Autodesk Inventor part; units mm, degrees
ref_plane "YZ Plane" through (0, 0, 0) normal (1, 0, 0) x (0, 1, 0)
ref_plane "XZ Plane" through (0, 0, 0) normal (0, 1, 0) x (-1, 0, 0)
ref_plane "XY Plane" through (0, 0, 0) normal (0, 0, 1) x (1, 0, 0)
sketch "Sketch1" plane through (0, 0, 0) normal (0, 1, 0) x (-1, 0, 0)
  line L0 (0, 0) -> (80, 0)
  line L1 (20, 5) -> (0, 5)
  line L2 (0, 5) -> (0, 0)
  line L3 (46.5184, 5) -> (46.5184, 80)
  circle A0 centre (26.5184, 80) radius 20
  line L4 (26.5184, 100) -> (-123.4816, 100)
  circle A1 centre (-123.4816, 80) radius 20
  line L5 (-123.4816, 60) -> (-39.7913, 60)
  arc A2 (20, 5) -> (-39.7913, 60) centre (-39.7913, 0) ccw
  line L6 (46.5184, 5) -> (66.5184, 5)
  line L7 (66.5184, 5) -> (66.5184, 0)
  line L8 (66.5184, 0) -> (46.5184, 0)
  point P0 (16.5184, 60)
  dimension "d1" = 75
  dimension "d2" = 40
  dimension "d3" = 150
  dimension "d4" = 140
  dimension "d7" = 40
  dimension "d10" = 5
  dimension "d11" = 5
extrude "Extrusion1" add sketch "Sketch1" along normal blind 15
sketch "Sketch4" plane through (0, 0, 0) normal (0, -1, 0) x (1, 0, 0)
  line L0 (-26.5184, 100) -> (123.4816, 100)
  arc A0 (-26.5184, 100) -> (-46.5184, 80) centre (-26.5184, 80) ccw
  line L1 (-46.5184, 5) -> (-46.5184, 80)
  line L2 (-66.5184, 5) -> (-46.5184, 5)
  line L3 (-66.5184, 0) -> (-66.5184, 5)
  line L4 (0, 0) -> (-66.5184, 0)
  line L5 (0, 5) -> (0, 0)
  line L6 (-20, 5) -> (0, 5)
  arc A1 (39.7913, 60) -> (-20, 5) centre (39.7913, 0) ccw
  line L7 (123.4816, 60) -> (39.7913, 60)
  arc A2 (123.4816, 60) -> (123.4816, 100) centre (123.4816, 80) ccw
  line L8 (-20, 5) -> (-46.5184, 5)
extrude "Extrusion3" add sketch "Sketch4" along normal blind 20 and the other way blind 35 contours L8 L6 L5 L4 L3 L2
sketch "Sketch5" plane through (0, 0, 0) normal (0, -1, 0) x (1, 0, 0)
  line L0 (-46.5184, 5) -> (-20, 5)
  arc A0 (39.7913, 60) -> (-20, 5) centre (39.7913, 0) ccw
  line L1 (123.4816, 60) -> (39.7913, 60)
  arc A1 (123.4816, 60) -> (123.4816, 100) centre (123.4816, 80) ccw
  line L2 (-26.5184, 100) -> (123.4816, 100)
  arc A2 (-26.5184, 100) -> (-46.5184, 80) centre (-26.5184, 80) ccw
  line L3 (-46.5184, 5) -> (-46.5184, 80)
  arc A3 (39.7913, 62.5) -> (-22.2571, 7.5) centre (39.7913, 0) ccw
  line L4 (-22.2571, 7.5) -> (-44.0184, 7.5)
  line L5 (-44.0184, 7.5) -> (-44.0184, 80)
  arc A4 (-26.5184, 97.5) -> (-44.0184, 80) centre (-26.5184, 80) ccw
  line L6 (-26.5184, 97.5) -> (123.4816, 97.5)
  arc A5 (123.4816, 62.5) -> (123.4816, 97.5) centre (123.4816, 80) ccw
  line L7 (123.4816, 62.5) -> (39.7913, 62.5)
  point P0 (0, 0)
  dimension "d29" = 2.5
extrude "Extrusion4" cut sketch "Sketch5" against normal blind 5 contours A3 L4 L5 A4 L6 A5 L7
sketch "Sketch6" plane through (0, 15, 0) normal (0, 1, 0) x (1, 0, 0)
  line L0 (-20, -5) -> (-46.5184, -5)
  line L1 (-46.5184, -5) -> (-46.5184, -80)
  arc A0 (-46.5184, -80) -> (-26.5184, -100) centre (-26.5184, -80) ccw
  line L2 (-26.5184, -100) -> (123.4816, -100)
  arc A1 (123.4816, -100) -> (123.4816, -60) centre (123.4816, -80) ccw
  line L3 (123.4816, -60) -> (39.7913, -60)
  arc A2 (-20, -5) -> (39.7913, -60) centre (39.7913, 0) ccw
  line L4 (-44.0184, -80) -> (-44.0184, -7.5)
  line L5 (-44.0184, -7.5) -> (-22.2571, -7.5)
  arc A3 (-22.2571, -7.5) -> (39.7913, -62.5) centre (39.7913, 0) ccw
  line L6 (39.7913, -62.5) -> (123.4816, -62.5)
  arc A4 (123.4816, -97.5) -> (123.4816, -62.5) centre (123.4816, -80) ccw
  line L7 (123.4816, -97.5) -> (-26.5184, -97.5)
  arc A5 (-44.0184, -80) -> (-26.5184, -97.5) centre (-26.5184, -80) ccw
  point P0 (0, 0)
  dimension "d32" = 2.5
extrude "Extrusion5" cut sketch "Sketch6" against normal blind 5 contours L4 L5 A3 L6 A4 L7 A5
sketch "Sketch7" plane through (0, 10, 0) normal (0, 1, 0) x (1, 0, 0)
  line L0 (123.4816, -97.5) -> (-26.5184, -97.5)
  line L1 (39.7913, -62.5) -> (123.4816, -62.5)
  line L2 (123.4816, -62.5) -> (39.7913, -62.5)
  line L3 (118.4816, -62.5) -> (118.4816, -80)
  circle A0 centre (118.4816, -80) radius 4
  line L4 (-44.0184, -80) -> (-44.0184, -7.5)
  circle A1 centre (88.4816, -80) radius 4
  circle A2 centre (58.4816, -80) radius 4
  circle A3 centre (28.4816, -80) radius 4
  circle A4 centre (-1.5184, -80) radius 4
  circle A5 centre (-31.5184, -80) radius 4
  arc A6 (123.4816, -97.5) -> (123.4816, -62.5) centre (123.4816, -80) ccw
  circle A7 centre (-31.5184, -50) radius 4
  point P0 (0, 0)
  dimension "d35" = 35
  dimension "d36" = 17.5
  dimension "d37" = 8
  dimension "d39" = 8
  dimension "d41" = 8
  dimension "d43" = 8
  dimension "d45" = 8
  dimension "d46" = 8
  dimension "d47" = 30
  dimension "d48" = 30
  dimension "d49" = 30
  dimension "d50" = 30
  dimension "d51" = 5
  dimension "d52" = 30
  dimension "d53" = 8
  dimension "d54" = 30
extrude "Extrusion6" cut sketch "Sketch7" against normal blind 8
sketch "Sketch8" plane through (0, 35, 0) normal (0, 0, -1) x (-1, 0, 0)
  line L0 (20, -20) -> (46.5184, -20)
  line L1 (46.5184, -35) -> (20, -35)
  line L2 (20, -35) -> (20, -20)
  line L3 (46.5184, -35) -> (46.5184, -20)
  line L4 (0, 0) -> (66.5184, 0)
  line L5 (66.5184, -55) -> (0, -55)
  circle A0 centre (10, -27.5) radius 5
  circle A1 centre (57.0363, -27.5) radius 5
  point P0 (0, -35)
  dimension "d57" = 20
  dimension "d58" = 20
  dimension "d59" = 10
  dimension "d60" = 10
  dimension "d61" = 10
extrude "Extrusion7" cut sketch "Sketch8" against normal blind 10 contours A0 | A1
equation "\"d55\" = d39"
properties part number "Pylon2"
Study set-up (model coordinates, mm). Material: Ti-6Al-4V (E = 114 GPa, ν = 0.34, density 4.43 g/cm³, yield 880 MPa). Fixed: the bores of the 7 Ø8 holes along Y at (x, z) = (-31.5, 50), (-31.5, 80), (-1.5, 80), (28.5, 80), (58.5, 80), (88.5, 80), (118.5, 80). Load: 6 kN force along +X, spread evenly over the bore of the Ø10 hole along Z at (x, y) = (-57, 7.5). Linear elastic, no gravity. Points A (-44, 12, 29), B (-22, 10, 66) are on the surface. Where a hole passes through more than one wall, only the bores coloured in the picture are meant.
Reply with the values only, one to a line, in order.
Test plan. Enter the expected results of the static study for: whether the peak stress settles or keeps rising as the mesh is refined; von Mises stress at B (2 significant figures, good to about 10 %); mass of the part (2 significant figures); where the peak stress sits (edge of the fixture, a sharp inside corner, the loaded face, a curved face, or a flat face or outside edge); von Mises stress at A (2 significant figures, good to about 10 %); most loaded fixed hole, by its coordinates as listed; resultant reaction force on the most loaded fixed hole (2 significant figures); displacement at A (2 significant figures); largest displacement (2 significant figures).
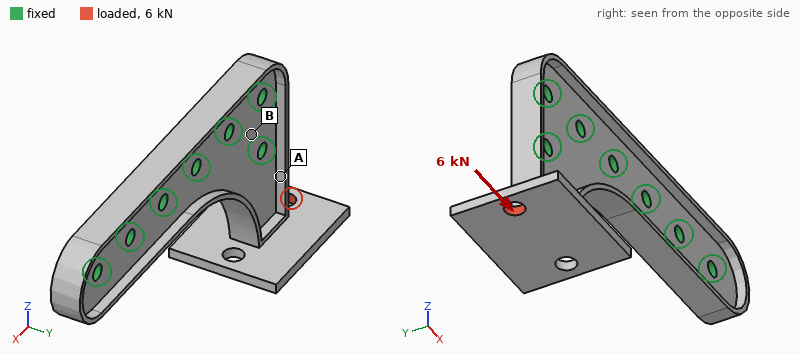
keeps rising
22 MPa
340 g
edge of the fixture
71 MPa
(-31.5, 50)
7.1 kN
0.048 mm
0.17 mm
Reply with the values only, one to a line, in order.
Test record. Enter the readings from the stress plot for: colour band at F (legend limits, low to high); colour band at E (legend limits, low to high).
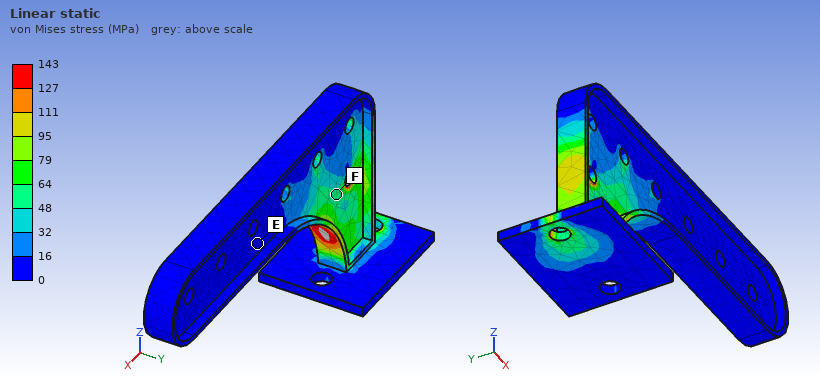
48 to 64 MPa
0 to 16 MPa
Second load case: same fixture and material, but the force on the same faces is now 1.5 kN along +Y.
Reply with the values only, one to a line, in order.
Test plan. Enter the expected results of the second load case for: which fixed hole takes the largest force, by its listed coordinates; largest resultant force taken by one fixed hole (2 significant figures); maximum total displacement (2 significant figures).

(-31.5, 50)
3.0 kN
0.92 mm
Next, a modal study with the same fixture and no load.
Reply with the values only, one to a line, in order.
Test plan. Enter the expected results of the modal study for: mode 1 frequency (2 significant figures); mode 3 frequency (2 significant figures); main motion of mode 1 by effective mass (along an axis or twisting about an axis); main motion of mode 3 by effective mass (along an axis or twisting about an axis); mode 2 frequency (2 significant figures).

890 Hz
3300 Hz
along Y
along X
1200 Hz
